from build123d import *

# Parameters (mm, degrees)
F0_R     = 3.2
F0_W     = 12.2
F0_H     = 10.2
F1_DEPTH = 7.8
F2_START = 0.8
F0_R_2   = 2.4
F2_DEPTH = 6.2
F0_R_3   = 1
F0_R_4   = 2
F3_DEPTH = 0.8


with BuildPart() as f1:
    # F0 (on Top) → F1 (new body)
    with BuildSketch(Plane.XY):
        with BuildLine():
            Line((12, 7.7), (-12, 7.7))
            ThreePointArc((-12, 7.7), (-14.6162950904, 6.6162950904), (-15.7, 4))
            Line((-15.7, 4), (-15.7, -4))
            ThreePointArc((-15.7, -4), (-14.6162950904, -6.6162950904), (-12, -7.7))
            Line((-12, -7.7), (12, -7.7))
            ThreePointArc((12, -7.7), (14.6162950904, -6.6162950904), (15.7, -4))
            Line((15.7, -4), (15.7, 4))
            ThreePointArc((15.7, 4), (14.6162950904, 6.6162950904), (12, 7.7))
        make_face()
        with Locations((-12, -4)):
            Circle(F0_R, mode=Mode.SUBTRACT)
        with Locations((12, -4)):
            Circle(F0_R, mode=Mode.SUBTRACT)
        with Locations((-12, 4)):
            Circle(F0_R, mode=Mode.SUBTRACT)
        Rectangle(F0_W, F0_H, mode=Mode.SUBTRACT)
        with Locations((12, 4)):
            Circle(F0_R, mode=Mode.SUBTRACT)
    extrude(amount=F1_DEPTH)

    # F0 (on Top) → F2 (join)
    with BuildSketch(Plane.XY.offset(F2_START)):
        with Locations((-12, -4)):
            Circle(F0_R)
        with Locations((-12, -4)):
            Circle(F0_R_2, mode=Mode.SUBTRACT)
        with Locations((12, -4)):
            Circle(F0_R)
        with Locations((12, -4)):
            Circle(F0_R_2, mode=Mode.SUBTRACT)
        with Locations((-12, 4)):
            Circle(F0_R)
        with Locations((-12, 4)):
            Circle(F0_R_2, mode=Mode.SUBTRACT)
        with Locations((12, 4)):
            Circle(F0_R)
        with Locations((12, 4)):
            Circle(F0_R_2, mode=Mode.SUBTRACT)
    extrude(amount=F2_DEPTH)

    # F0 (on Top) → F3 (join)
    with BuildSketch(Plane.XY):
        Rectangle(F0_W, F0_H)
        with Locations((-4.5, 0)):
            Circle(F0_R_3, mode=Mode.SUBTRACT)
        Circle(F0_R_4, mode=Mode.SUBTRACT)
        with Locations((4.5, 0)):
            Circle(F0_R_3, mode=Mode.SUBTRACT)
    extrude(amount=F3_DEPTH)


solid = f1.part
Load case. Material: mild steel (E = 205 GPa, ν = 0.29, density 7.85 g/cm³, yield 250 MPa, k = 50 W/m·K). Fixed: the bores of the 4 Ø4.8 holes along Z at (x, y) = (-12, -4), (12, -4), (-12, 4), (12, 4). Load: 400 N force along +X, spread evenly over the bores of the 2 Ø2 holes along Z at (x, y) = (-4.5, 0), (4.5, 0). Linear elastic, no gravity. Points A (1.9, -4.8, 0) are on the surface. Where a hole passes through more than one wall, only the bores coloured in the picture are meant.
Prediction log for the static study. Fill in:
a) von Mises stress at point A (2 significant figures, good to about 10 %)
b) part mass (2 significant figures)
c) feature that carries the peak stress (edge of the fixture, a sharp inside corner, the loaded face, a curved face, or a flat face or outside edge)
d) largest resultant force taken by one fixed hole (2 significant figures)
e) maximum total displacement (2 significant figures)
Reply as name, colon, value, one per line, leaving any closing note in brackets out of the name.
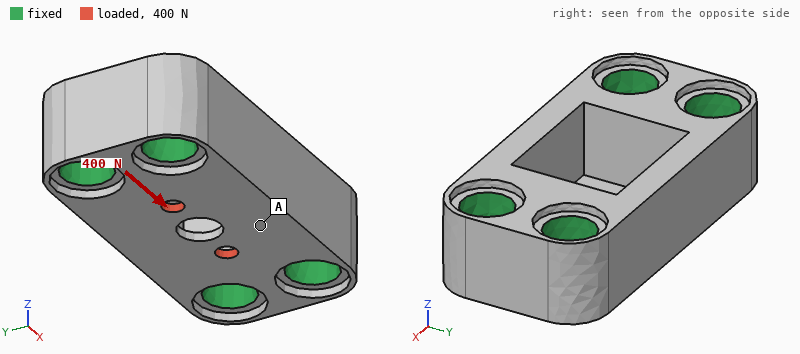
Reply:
von Mises stress at point A: 7.6 MPa
part mass: 17 g
feature that carries the peak stress: the loaded face
largest resultant force taken by one fixed hole: 110 N
maximum total displacement: 1.1 µm
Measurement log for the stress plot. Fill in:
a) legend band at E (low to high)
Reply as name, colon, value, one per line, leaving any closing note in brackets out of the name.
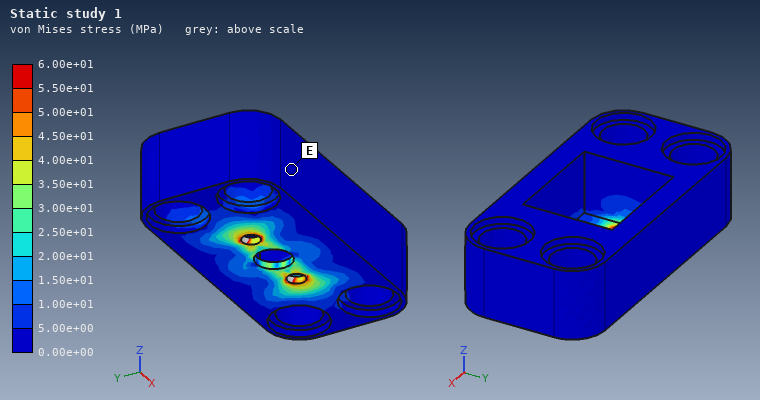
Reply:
legend band at E: 0.00e+00 to 5.00e+00 MPa
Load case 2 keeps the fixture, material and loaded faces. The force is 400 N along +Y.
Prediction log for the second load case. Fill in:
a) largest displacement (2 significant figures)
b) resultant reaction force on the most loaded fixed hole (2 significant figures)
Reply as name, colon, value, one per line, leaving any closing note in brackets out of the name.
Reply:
largest displacement: 1.1 µm
resultant reaction force on the most loaded fixed hole: 130 N
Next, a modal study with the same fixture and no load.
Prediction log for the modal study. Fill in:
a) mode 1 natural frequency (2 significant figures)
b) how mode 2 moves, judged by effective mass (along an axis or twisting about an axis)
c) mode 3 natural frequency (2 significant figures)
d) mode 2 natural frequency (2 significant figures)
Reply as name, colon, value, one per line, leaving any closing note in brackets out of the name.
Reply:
mode 1 natural frequency: 50 kHz
how mode 2 moves, judged by effective mass: along Y
mode 3 natural frequency: 59 kHz
mode 2 natural frequency: 55 kHz
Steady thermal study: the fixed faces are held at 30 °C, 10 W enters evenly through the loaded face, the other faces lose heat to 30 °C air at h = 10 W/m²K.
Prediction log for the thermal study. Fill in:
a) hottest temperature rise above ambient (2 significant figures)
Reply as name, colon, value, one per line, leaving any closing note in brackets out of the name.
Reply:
hottest temperature rise above ambient: 46 K
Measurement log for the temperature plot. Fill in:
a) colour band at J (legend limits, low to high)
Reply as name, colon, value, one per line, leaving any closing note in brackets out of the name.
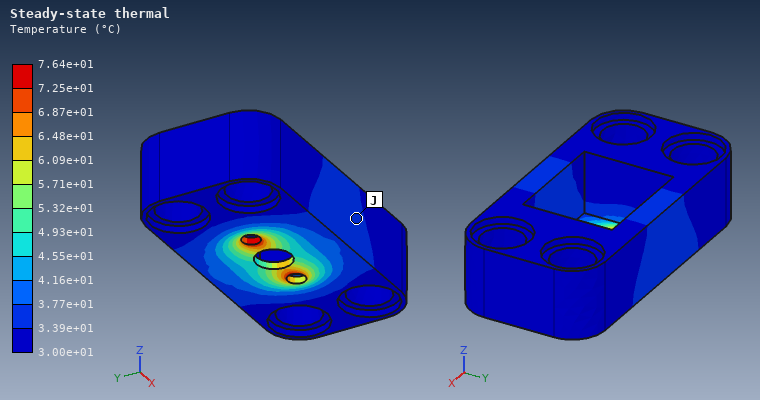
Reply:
colour band at J: 3.39e+01 to 3.77e+01 °C
